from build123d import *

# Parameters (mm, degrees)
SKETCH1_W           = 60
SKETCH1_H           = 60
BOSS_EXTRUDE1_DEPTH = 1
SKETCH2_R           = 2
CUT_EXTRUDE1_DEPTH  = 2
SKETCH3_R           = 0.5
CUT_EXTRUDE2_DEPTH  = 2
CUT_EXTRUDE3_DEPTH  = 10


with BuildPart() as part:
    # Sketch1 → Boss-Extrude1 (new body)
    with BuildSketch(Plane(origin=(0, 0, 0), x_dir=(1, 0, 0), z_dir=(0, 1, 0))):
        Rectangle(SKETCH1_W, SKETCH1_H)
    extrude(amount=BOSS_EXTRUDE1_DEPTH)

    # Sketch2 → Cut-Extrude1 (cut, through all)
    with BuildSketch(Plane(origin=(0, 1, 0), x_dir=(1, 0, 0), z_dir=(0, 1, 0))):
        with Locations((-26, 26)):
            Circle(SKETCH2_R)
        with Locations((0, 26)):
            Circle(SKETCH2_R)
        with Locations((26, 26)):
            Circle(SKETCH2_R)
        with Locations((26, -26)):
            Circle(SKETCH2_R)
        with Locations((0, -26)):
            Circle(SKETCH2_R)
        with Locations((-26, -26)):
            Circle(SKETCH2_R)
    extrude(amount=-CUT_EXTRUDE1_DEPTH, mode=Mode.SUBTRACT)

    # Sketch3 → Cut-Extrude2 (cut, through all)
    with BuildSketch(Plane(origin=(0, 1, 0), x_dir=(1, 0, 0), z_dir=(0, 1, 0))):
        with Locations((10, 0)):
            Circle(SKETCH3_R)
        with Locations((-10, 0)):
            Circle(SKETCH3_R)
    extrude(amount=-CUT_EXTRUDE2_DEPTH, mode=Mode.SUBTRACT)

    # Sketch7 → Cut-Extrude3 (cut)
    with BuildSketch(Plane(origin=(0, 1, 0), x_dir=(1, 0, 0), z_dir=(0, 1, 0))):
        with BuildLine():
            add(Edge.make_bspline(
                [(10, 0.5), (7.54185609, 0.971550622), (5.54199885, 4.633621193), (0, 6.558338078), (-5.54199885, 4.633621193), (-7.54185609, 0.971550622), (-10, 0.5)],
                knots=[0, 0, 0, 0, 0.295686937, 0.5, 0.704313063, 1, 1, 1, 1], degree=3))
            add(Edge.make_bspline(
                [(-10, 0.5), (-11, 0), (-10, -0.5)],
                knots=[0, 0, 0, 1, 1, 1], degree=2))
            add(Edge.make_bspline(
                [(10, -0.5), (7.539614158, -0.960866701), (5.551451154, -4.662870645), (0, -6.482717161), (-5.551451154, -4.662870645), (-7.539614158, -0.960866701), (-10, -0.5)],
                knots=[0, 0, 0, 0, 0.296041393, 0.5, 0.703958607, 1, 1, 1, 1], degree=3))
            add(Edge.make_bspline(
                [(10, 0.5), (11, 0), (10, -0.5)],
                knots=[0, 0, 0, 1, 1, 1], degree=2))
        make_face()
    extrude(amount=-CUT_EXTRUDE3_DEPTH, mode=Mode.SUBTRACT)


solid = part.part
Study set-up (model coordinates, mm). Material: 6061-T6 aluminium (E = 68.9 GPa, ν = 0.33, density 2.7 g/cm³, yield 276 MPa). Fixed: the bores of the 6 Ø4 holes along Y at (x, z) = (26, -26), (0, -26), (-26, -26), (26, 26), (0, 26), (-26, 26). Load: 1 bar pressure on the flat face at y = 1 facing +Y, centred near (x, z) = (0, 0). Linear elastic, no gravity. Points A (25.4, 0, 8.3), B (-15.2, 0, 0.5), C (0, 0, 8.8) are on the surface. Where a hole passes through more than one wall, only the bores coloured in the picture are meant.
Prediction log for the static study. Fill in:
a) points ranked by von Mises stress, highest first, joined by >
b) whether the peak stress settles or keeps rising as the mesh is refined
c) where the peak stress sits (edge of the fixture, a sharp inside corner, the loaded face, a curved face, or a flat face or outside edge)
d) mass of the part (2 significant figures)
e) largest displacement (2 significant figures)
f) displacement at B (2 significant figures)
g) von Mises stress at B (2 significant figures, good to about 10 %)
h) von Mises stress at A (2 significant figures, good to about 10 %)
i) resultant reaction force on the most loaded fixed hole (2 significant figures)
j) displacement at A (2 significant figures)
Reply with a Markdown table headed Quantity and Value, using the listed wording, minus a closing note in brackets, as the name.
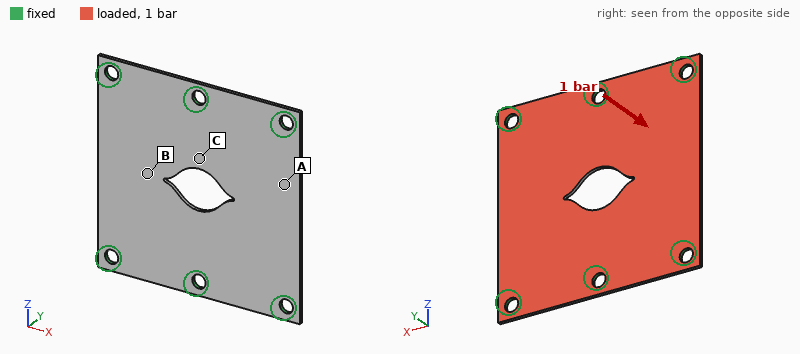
| Quantity | Value |
|---|---|
| points ranked by von Mises stress, highest first, joined by > | B > A > C |
| whether the peak stress settles or keeps rising as the mesh is refined | keeps rising |
| where the peak stress sits | edge of the fixture |
| mass of the part | 9.1 g |
| largest displacement | 0.37 mm |
| displacement at B | 0.33 mm |
| von Mises stress at B | 74 MPa |
| von Mises stress at A | 45 MPa |
| resultant reaction force on the most loaded fixed hole | 73 N |
| displacement at A | 0.24 mm |
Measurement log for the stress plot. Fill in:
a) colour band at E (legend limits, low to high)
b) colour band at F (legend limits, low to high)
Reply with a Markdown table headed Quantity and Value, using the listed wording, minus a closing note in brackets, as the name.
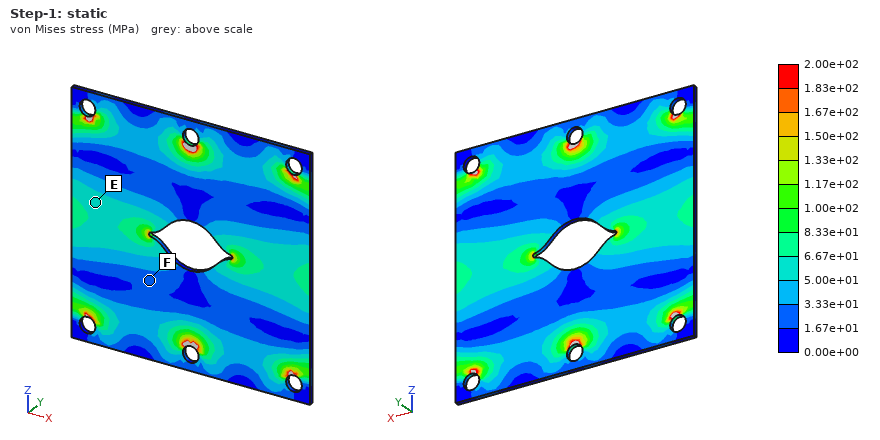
| Quantity | Value |
|---|---|
| colour band at E | 5.00e+01 to 6.67e+01 MPa |
| colour band at F | 1.67e+01 to 3.33e+01 MPa |
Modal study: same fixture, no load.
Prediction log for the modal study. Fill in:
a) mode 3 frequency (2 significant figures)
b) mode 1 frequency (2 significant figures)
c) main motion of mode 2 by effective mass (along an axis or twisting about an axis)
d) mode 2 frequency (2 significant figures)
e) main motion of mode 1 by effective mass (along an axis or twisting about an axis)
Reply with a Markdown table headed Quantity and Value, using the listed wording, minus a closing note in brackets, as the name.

| Quantity | Value |
|---|---|
| mode 3 frequency | 3600 Hz |
| mode 1 frequency | 2000 Hz |
| main motion of mode 2 by effective mass | twisting about Z |
| mode 2 frequency | 2300 Hz |
| main motion of mode 1 by effective mass | along Y |
